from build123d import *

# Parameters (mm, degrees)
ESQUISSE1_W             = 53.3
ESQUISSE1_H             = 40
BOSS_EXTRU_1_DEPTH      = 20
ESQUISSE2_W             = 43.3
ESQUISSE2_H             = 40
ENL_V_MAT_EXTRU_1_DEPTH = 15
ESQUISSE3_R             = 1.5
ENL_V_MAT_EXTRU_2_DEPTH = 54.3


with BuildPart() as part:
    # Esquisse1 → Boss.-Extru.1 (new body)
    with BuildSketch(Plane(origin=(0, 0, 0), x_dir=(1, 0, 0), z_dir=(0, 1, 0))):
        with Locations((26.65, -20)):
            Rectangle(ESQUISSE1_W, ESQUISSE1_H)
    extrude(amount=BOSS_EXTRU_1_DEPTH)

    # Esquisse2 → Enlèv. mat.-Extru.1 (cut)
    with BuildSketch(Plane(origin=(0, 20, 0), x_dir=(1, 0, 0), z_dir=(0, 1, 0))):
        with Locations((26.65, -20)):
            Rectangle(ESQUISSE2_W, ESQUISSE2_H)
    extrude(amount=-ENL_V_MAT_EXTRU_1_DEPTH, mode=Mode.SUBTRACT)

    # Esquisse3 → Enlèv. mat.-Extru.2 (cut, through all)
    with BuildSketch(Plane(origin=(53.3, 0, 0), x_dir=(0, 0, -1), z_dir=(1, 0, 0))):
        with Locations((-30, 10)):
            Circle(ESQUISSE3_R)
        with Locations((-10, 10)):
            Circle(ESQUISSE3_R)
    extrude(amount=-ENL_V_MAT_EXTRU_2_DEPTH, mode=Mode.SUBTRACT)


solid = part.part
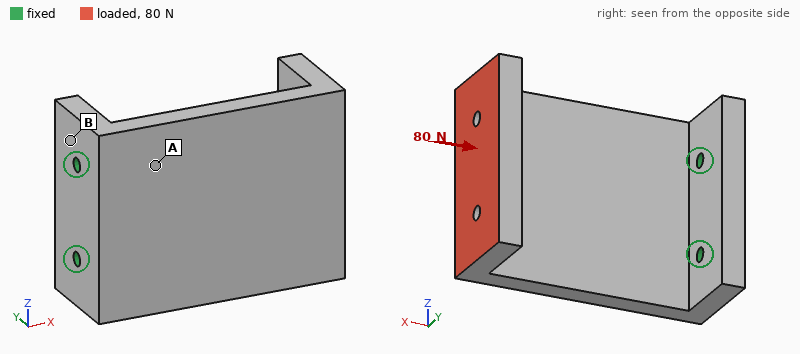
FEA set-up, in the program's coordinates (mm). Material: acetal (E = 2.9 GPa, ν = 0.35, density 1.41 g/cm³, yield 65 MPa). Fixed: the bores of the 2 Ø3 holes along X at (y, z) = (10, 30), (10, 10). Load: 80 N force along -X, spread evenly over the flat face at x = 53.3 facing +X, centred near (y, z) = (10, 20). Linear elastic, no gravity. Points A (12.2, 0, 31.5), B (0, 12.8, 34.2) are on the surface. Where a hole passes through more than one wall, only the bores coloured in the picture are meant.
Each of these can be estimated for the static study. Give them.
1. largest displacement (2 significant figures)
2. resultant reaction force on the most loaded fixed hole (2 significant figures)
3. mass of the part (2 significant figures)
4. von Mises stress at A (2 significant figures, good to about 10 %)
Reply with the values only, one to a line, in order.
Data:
0.79 mm
40 N
23 g
2.9 MPa
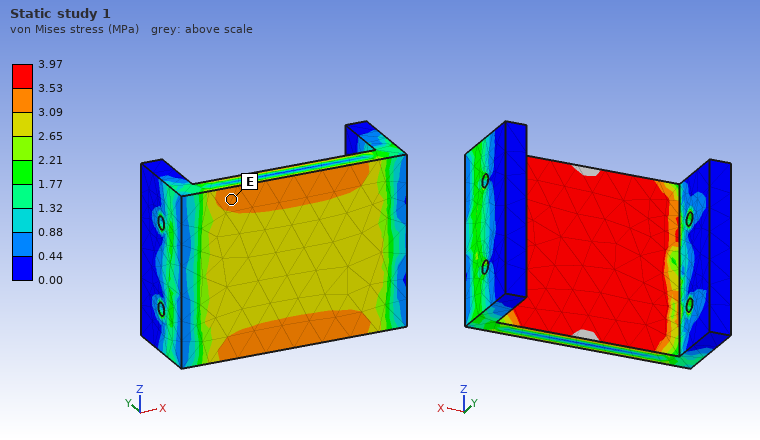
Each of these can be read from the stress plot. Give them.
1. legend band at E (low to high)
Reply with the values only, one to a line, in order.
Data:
3.09 to 3.53 MPa
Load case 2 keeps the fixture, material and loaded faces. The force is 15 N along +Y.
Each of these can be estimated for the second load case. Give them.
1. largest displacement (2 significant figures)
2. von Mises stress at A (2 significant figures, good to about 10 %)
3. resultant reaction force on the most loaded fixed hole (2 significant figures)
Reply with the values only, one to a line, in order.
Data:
0.80 mm
3.4 MPa
8.3 N
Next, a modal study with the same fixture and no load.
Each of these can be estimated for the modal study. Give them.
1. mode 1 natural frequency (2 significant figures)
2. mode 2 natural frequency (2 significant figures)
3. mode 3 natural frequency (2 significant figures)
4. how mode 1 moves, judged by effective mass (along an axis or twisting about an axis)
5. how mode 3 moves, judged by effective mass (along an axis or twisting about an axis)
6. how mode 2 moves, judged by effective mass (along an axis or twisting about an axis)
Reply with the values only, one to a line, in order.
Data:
260 Hz
660 Hz
1100 Hz
along Y
along Z
along Z
